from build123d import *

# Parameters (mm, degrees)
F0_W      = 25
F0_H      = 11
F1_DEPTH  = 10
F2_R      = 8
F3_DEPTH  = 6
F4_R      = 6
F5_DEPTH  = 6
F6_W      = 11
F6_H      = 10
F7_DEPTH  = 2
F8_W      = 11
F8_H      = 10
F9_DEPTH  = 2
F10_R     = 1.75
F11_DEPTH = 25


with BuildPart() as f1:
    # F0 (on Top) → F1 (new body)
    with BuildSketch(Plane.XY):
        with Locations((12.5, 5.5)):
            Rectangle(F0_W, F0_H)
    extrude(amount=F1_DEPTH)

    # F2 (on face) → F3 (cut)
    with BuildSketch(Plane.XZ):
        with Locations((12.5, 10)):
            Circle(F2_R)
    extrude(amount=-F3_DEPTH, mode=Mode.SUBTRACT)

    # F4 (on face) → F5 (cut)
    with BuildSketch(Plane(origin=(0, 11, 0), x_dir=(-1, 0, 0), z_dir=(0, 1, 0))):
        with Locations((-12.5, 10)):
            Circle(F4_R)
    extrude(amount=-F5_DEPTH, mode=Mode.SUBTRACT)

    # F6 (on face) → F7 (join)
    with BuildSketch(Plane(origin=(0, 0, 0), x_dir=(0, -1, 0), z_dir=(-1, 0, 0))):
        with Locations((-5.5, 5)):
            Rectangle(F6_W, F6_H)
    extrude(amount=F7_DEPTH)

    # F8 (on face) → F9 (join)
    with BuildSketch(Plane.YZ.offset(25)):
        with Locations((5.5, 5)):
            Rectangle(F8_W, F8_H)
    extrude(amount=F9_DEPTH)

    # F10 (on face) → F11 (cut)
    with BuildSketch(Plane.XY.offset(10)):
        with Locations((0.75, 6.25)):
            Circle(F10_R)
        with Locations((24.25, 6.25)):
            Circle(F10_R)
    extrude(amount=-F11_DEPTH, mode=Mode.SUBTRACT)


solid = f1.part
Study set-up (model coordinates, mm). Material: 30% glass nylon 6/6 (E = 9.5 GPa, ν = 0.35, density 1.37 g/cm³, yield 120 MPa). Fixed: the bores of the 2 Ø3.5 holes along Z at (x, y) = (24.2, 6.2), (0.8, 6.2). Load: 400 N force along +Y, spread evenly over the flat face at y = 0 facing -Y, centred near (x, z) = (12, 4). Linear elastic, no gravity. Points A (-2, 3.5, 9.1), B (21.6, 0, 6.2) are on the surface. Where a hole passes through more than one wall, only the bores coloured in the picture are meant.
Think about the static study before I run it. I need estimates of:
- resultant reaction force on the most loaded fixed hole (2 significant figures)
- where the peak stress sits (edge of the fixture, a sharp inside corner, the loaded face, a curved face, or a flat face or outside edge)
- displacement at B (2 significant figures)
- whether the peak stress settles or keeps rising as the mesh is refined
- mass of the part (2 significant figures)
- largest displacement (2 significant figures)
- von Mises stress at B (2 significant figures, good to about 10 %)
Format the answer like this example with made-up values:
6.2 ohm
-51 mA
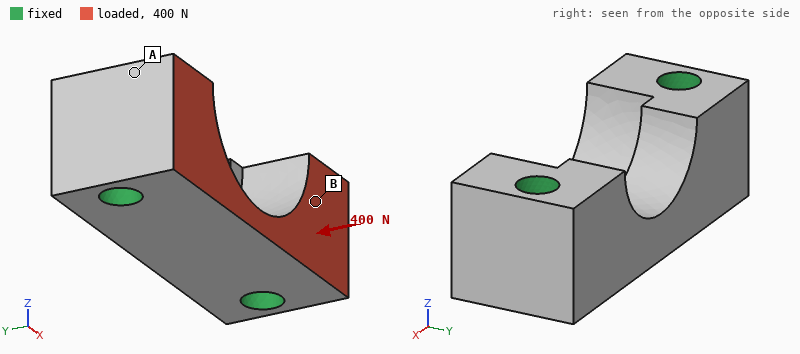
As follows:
200 N
edge of the fixture
2.7 µm
keeps rising
2.9 g
6.9 µm
2.8 MPa
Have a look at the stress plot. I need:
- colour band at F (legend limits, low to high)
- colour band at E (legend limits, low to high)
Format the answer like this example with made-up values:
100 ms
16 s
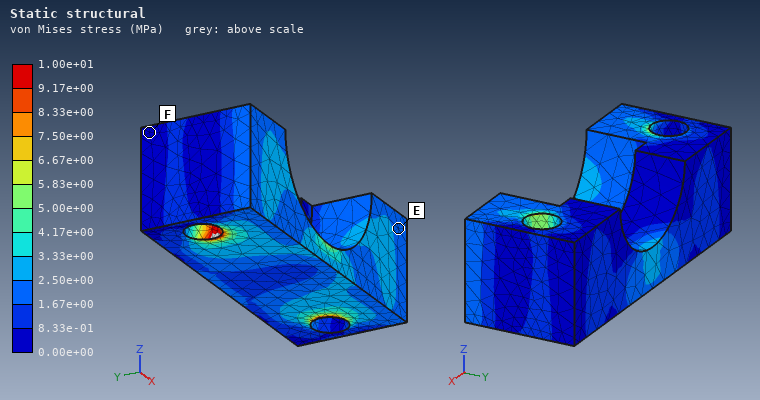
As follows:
0.00e+00 to 8.33e-01 MPa
1.67e+00 to 2.50e+00 MPa
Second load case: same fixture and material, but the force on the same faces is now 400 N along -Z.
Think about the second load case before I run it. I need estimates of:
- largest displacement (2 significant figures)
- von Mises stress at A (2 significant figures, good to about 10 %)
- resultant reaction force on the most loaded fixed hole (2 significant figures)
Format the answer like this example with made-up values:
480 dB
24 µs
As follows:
20 µm
2.9 MPa
200 N
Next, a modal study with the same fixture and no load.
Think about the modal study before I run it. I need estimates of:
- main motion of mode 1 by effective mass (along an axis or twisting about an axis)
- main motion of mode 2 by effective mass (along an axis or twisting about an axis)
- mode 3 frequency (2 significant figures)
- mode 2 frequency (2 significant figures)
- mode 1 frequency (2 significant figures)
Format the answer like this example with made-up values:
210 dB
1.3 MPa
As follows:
along Y
along Z
42 kHz
33 kHz
27 kHz
